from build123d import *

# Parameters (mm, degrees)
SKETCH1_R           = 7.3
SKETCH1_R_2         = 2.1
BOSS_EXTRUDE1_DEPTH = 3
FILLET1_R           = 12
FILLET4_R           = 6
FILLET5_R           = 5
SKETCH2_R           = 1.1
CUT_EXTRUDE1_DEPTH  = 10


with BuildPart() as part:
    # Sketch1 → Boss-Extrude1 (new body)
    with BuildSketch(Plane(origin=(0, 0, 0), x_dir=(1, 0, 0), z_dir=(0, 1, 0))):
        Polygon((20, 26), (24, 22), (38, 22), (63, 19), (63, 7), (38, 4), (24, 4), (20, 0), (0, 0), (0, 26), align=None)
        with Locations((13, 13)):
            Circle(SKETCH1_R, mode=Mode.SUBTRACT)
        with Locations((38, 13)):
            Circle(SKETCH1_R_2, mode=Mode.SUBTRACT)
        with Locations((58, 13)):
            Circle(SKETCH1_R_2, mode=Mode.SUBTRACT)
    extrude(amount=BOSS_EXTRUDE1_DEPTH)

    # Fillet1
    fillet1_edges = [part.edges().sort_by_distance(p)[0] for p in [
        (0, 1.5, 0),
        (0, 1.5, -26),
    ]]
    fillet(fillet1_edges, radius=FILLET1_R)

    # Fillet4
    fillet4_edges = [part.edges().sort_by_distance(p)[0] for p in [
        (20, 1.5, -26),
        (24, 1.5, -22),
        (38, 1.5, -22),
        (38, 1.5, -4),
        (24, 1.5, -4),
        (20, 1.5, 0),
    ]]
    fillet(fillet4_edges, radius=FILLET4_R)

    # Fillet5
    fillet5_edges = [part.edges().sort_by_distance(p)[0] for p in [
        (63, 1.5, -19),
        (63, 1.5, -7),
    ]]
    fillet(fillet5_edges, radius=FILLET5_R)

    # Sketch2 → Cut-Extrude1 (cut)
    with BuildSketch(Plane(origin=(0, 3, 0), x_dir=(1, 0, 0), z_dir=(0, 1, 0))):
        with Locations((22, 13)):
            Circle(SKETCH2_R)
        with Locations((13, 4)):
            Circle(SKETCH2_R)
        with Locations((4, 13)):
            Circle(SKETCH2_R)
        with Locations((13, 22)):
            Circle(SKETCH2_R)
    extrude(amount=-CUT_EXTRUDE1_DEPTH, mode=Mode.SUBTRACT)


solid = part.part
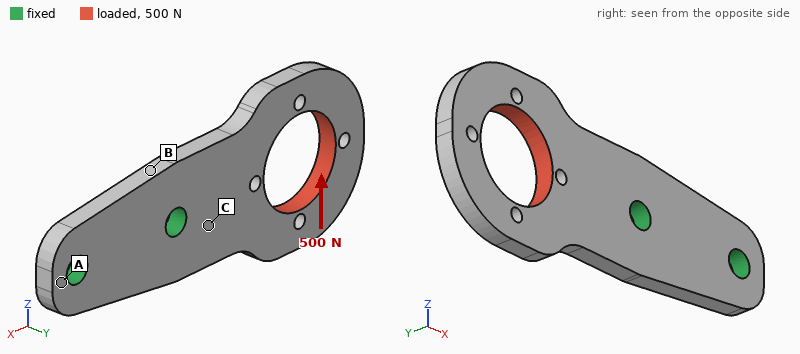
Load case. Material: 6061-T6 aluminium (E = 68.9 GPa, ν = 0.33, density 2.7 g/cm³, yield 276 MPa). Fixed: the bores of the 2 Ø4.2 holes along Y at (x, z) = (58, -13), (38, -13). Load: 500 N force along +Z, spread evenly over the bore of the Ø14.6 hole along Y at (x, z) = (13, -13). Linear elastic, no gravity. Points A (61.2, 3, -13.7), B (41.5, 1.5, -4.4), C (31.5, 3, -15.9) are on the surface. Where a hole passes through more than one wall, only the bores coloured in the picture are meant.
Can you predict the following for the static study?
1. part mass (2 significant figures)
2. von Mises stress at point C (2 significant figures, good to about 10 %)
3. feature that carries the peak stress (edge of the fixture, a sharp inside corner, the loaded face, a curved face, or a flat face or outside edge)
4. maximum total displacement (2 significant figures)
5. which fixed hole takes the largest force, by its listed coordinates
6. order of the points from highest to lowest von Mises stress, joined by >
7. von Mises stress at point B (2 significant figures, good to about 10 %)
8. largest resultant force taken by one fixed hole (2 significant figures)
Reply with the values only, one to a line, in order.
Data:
7.7 g
28 MPa
edge of the fixture
0.12 mm
(38, -13)
B > C > A
55 MPa
900 N
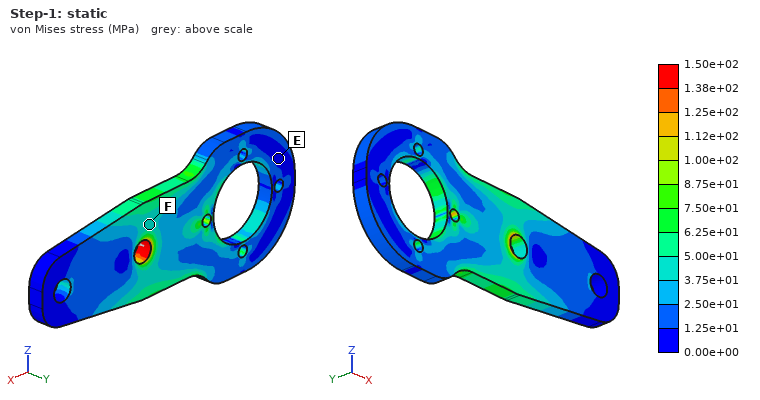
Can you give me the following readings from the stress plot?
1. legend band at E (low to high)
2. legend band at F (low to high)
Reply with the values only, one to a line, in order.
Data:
0.00e+00 to 1.25e+01 MPa
3.75e+01 to 5.00e+01 MPa
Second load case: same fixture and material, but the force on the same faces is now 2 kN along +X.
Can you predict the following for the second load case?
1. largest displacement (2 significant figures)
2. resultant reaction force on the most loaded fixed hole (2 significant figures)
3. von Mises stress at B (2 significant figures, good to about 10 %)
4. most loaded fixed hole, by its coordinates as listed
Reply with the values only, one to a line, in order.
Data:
42 µm
1.7 kN
21 MPa
(38, -13)
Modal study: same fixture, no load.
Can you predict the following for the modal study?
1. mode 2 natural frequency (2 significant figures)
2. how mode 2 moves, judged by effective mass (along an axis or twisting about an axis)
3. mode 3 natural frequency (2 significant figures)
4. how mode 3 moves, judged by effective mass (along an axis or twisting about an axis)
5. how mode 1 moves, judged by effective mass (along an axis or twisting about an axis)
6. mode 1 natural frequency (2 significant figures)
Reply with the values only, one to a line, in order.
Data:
4700 Hz
twisting about X
6500 Hz
along Z
along Y
1900 Hz
